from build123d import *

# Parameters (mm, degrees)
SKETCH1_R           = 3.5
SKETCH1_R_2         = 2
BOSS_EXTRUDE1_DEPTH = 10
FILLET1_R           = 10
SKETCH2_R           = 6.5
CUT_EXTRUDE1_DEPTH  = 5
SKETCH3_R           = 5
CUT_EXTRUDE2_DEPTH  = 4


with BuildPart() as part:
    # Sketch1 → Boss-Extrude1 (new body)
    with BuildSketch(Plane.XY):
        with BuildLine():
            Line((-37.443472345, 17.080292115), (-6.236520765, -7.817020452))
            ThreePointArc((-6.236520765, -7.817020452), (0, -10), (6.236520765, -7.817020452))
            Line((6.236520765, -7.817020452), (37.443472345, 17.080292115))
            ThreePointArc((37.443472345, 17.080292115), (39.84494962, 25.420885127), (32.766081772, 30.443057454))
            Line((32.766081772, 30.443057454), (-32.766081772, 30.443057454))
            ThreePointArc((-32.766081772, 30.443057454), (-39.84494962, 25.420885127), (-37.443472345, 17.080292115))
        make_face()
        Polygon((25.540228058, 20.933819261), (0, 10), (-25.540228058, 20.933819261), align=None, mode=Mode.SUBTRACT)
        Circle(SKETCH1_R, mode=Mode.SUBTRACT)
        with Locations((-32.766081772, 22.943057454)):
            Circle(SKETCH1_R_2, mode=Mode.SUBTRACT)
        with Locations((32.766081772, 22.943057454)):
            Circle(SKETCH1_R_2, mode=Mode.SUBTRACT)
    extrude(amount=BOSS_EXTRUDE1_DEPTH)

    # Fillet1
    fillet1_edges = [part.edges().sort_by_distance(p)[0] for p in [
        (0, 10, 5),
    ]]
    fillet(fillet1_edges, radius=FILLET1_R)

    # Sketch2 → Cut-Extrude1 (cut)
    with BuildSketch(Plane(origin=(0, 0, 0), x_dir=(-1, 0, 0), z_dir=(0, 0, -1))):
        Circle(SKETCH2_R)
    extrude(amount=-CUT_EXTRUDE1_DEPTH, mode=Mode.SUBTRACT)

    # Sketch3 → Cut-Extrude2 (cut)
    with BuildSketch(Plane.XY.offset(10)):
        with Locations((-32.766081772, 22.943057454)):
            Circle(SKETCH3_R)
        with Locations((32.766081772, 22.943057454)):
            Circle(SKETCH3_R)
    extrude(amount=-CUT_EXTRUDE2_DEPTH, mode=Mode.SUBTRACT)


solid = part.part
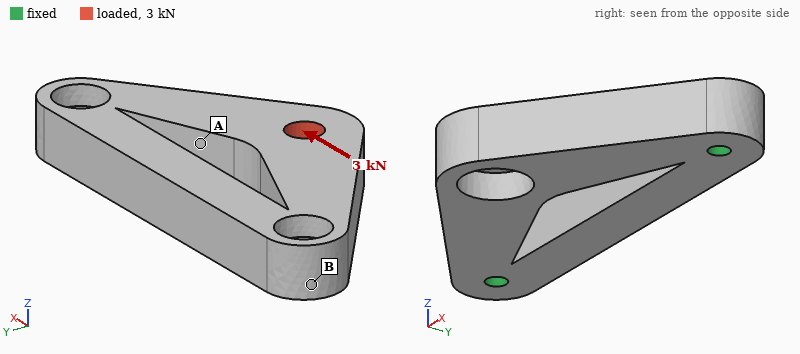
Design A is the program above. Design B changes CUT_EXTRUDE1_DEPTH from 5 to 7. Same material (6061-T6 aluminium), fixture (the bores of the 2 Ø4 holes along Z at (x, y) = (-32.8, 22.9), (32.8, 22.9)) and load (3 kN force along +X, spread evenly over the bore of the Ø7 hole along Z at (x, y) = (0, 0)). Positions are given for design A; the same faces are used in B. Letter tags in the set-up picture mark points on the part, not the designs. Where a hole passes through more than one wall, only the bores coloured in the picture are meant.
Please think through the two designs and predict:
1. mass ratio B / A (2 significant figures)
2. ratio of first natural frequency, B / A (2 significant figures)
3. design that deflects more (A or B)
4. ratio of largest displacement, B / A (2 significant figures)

0.99
1.0
B
1.2
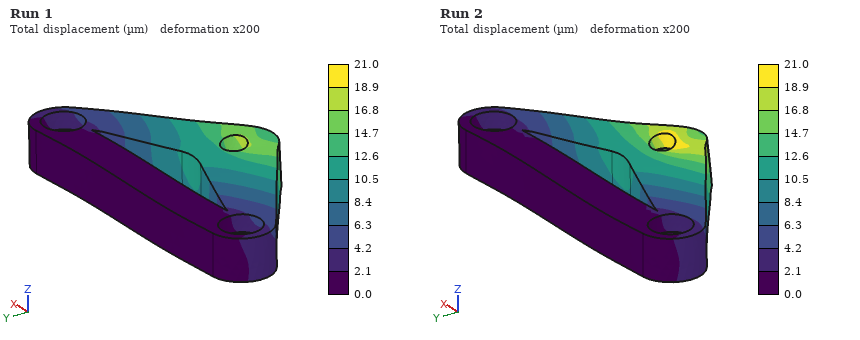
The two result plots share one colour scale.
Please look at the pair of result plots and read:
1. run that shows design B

Run 2
